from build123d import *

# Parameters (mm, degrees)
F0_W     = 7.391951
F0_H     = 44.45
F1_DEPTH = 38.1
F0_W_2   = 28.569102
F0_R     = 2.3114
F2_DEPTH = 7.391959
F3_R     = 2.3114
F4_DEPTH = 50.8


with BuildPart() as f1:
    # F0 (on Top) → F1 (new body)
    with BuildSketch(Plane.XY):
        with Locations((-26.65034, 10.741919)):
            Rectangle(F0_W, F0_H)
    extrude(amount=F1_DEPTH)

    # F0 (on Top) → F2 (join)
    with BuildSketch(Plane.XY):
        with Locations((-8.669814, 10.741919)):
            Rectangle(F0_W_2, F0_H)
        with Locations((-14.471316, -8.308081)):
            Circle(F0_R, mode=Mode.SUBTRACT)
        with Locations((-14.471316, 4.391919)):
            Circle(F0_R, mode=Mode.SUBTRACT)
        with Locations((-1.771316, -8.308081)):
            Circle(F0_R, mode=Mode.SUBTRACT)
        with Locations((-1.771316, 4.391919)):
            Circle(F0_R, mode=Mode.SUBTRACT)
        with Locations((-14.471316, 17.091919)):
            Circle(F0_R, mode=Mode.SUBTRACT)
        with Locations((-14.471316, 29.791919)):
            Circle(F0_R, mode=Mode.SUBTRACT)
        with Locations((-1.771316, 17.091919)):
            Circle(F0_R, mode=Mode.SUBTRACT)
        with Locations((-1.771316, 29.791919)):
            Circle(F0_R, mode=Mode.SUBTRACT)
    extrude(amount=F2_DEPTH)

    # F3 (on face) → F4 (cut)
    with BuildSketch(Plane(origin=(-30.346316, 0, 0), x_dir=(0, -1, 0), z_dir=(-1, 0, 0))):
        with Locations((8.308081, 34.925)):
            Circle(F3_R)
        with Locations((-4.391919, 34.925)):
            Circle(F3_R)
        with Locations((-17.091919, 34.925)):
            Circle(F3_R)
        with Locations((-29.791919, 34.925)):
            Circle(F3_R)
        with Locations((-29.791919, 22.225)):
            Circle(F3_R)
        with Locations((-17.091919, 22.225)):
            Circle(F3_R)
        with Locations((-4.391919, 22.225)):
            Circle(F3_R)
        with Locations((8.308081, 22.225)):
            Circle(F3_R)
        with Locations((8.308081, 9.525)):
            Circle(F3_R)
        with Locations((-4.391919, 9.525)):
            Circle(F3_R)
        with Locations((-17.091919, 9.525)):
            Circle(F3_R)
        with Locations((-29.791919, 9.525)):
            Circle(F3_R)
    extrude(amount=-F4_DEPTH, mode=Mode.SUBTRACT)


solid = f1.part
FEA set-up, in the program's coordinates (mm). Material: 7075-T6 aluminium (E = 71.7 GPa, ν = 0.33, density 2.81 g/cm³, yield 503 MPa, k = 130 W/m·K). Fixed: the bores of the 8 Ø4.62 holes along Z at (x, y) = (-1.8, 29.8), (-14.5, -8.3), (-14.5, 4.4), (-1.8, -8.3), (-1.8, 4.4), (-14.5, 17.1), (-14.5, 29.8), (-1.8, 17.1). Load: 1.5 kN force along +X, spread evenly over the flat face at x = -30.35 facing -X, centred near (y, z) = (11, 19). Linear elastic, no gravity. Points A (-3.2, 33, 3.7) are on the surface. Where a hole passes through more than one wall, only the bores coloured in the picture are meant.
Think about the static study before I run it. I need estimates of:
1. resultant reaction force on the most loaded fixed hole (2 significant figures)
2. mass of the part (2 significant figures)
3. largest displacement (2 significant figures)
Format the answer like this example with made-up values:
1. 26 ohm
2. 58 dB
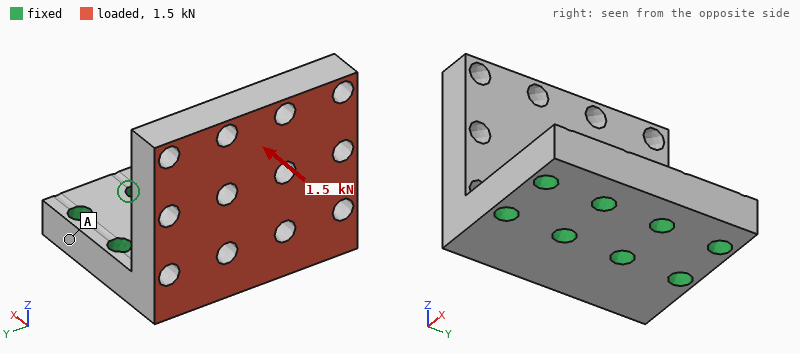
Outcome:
1. 470 N
2. 55 g
3. 0.15 mm
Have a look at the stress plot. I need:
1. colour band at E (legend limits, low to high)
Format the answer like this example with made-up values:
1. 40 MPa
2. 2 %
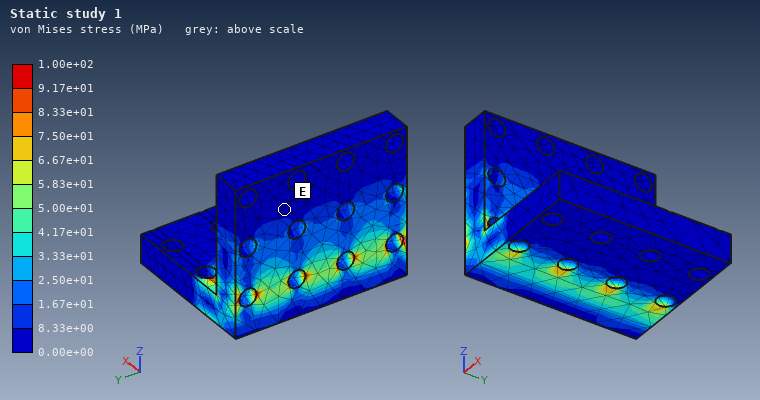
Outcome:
1. 0.00e+00 to 8.33e+00 MPa
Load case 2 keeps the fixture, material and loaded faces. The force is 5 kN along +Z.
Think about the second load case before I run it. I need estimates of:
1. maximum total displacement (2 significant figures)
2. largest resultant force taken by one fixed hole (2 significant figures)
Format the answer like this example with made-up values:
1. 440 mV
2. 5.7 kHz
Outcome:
1. 0.25 mm
2. 1.7 kN
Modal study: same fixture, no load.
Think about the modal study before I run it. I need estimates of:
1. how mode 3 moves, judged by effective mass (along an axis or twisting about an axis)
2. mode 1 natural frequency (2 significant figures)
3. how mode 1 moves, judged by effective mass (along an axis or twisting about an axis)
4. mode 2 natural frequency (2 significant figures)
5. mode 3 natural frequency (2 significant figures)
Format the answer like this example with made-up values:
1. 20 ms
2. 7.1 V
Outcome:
1. along Y
2. 3600 Hz
3. along X
4. 7200 Hz
5. 9600 Hz
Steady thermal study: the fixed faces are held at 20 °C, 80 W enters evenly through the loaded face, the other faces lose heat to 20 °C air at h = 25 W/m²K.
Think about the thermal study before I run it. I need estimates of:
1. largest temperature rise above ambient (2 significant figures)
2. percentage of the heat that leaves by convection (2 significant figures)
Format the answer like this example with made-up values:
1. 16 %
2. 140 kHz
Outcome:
1. 50 K
2. 4.5 %
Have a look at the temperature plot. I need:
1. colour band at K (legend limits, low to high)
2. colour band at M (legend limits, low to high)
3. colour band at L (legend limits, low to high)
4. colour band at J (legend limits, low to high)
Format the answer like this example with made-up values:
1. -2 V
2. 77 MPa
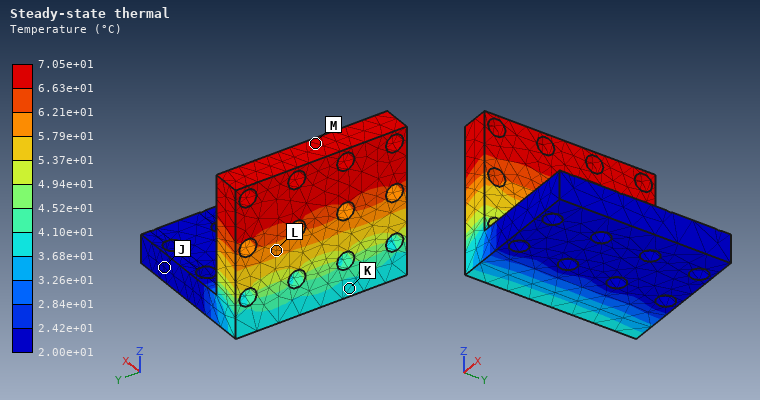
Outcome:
1. 3.68e+01 to 4.10e+01 °C
2. 6.63e+01 to 7.05e+01 °C
3. 5.79e+01 to 6.21e+01 °C
4. 2.00e+01 to 2.42e+01 °C
